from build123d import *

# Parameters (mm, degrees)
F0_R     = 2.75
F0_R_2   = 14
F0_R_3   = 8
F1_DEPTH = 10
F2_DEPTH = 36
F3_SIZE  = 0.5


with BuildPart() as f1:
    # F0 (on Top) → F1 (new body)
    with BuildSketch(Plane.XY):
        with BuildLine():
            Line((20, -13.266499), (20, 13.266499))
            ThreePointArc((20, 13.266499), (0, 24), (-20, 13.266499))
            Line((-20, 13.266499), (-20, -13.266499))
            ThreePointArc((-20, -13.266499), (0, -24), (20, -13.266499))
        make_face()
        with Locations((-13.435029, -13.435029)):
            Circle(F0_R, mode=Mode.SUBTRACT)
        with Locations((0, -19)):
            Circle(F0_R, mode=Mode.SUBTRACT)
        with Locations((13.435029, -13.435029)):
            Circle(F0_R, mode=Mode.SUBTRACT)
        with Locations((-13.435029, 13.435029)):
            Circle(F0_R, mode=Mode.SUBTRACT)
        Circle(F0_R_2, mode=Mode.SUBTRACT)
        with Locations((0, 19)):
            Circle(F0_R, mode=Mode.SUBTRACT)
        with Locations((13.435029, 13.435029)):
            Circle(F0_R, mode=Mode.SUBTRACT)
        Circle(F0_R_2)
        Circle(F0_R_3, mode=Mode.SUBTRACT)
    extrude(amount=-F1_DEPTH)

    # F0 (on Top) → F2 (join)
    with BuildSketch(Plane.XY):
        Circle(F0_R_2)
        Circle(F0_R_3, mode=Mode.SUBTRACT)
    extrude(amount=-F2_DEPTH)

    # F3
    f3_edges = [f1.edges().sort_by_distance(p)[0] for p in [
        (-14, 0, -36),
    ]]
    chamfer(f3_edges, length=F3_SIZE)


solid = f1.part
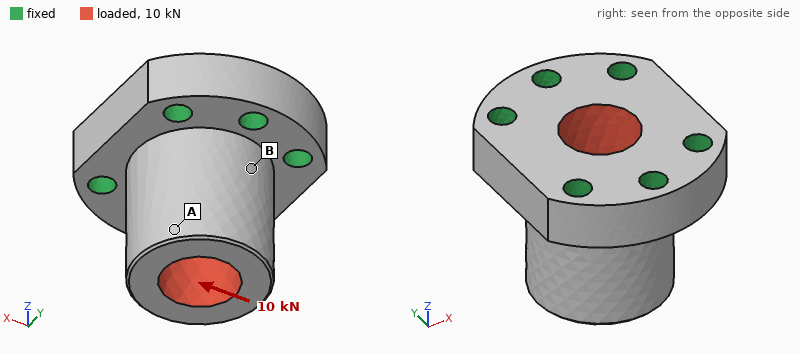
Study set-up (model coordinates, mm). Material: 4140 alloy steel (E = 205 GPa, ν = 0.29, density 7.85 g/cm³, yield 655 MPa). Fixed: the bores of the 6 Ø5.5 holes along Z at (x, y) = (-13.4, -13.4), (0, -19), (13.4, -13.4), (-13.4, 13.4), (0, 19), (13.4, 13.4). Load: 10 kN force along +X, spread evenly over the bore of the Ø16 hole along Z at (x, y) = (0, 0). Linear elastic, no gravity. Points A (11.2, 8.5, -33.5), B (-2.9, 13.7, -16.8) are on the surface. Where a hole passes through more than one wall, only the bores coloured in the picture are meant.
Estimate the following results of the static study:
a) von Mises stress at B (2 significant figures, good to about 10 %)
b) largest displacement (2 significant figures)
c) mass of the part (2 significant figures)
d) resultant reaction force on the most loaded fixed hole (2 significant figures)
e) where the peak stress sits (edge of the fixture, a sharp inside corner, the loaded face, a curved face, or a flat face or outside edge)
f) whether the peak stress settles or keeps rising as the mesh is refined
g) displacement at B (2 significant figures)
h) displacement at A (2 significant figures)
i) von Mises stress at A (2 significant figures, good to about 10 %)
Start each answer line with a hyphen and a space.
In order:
- 27 MPa
- 14 µm
- 190 g
- 3.2 kN
- edge of the fixture
- keeps rising
- 4.6 µm
- 13 µm
- 8.4 MPa
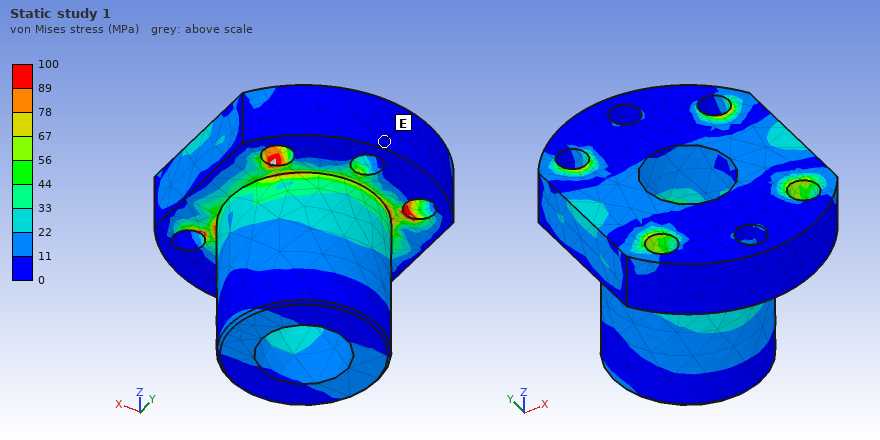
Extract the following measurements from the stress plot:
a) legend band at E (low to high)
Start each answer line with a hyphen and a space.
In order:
- 0 to 11 MPa
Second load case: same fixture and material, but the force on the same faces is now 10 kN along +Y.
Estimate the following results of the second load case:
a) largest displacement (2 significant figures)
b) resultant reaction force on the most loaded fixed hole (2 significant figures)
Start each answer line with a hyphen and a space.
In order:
- 12 µm
- 2.8 kN
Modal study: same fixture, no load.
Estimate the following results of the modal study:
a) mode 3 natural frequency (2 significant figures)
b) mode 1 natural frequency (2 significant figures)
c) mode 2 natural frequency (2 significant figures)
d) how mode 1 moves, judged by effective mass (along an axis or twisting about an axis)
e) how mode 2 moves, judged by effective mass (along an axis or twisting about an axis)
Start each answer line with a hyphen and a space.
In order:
- 27 kHz
- 15 kHz
- 16 kHz
- along X
- along Y
